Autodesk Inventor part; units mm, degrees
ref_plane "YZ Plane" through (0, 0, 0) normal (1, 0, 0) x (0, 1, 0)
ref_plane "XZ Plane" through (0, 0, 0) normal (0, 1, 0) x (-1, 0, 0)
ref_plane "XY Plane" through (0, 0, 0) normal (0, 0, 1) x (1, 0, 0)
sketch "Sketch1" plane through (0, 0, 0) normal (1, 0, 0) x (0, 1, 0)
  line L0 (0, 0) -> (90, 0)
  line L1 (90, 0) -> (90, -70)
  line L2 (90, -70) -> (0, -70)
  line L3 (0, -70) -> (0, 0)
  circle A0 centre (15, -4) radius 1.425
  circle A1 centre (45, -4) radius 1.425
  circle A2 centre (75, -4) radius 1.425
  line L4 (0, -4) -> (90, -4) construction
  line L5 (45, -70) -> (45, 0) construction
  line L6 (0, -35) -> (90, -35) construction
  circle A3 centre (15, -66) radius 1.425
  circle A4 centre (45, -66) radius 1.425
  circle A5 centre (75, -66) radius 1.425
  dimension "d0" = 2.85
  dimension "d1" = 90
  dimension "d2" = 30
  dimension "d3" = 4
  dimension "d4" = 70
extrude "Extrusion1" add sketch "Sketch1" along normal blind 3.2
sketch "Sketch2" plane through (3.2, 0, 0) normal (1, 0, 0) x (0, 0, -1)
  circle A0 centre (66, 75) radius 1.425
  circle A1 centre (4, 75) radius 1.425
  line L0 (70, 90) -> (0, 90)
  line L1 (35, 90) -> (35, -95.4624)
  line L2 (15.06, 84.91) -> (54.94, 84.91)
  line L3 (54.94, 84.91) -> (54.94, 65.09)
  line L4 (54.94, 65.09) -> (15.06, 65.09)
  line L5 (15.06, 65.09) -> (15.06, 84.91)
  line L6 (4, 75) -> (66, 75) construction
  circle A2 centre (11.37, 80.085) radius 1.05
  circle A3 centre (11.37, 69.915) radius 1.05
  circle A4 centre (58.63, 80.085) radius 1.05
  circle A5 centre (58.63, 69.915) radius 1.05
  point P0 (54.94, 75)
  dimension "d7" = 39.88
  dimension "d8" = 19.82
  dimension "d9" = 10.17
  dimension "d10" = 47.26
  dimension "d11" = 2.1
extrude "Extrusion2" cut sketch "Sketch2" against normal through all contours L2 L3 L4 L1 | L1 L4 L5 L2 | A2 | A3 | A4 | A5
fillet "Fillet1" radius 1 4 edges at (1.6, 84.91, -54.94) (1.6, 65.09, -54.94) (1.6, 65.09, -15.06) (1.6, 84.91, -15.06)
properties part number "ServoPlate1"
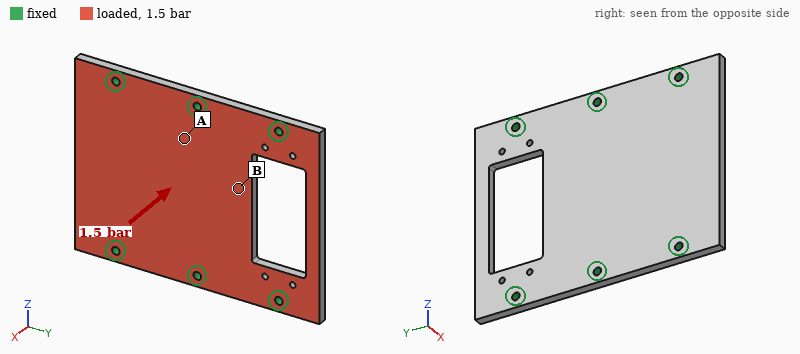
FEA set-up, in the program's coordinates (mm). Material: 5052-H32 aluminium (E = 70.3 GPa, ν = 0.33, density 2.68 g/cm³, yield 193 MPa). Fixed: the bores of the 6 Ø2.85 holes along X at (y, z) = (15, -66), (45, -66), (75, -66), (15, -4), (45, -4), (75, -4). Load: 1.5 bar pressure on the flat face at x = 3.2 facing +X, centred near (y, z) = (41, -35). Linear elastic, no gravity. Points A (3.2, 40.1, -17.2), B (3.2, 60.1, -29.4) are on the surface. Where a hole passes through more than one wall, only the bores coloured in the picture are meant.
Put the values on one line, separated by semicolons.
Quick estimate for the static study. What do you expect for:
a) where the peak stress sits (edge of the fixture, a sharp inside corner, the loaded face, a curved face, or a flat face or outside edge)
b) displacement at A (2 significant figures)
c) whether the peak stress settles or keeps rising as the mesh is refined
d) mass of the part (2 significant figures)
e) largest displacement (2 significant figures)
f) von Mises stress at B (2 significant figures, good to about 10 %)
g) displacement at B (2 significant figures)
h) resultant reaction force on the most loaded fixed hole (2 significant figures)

edge of the fixture; 19 µm; keeps rising; 47 g; 51 µm; 14 MPa; 35 µm; 160 N
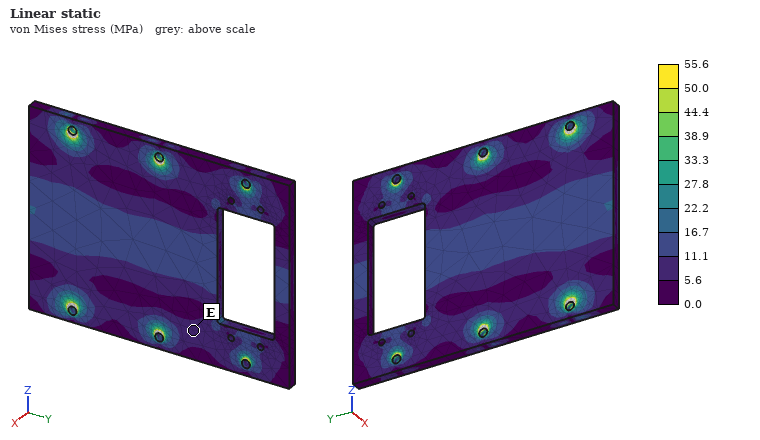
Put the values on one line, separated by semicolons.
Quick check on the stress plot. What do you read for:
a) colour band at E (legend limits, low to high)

5.6 to 11.1 MPa
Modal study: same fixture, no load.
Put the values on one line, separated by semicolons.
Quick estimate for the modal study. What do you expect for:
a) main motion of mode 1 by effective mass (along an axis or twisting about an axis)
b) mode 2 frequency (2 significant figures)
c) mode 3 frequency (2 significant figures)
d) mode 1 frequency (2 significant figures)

along X; 4300 Hz; 4500 Hz; 3700 Hz
